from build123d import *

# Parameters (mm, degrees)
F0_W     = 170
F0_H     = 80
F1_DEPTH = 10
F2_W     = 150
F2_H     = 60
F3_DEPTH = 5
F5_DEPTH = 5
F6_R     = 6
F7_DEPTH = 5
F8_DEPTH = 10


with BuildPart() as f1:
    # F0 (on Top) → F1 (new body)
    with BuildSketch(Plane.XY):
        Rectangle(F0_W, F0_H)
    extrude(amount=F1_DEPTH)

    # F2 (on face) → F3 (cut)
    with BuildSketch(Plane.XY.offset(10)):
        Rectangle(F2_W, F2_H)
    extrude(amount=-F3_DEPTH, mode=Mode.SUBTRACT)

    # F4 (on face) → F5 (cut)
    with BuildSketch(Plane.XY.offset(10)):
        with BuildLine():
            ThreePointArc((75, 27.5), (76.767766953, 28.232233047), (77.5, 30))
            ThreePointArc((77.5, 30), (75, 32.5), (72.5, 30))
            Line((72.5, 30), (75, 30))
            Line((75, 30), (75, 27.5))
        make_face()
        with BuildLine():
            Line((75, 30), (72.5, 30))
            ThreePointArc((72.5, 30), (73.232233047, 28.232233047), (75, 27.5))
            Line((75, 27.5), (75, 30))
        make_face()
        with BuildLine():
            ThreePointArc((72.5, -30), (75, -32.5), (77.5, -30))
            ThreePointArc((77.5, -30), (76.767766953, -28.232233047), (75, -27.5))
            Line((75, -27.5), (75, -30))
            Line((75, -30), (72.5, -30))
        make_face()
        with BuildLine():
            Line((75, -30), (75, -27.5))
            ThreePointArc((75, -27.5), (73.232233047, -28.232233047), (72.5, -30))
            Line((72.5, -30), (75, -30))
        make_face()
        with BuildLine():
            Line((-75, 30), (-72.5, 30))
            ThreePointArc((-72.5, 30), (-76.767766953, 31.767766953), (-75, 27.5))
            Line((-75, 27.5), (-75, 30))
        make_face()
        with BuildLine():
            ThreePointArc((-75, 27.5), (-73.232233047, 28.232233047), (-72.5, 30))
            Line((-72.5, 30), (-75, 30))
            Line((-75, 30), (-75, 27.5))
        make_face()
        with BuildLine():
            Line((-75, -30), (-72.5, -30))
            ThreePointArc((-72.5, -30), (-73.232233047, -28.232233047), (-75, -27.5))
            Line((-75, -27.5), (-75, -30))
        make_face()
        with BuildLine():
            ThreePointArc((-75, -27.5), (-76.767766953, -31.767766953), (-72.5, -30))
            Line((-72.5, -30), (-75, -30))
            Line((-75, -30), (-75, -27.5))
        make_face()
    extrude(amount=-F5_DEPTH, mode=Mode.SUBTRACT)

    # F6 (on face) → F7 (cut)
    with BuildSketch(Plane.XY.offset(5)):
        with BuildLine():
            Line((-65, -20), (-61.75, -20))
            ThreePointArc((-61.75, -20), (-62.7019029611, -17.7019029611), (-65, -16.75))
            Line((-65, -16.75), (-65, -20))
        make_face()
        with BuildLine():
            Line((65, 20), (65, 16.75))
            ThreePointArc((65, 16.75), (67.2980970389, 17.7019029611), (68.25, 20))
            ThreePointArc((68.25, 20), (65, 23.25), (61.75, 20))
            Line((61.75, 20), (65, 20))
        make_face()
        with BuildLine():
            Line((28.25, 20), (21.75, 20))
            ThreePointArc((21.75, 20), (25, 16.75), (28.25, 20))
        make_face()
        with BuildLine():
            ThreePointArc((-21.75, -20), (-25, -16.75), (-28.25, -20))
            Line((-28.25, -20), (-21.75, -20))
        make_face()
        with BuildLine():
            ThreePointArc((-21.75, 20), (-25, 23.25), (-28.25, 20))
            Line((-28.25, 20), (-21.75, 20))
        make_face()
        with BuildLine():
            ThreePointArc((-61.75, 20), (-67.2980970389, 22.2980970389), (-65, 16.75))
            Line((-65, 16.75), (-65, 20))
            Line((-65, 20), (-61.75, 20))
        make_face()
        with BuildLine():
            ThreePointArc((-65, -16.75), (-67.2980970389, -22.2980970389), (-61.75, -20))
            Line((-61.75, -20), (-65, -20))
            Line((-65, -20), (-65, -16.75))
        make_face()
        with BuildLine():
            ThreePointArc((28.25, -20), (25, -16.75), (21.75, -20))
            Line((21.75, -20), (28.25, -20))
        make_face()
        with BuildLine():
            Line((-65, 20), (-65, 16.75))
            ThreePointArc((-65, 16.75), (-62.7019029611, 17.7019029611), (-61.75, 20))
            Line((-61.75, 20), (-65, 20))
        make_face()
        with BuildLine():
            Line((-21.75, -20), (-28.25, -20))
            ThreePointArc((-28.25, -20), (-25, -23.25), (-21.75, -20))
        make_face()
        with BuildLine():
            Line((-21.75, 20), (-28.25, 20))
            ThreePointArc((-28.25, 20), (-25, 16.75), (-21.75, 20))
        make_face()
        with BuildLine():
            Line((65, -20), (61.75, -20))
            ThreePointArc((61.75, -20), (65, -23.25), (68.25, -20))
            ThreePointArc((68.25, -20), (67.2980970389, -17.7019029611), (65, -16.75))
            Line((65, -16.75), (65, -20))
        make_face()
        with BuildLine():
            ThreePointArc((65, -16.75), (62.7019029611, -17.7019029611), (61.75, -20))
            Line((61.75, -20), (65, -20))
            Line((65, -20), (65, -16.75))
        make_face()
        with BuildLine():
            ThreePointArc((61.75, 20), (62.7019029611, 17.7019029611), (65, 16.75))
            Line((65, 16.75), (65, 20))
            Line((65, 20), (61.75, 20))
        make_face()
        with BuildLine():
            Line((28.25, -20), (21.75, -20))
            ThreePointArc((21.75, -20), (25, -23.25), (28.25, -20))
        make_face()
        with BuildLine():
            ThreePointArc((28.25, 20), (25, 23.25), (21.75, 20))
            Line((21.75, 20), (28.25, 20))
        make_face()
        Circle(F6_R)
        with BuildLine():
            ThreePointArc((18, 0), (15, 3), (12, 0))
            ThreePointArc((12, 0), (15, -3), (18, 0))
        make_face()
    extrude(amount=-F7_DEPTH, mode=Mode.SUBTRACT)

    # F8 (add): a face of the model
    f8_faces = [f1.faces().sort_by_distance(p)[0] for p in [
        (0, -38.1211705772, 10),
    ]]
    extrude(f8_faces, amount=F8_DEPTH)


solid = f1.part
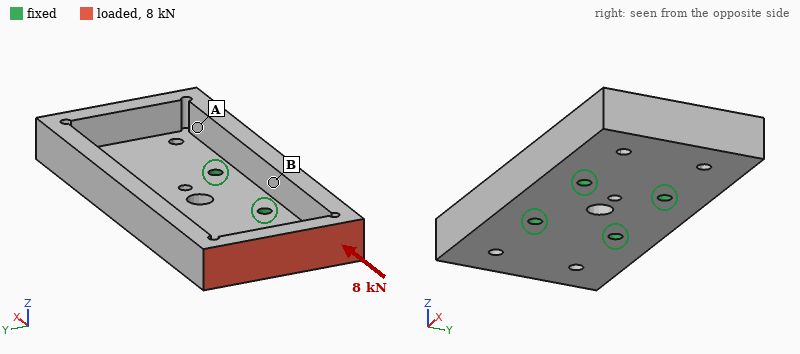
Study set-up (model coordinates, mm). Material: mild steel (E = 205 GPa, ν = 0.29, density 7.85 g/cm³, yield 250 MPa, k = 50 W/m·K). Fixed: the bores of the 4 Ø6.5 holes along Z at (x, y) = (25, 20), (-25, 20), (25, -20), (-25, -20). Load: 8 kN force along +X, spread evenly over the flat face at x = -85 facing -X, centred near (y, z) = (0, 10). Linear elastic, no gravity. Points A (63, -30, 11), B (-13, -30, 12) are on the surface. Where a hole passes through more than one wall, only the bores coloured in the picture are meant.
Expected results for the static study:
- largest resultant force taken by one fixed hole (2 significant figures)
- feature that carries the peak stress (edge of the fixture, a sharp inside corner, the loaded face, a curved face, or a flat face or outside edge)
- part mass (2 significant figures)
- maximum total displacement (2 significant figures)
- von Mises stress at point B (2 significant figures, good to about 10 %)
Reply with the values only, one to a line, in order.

2.7 kN
a curved face
1.1 kg
47 µm
14 MPa
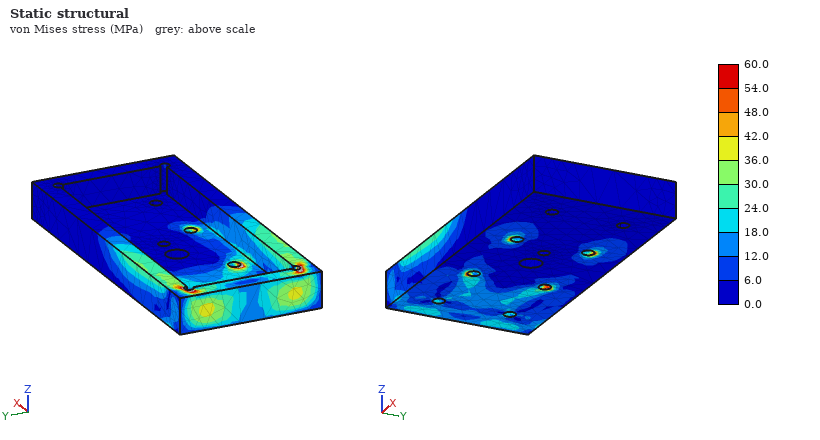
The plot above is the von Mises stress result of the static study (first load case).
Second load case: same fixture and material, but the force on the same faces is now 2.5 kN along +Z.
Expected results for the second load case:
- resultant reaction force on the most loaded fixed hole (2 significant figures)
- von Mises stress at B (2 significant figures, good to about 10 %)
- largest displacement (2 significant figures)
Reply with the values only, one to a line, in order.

3.1 kN
37 MPa
0.11 mm
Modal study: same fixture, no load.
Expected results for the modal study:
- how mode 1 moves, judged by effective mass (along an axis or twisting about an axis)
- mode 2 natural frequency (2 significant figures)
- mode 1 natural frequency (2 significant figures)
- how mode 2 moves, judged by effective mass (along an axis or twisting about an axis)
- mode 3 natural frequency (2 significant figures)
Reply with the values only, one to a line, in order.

twisting about Y
2100 Hz
1700 Hz
along Z
2300 Hz
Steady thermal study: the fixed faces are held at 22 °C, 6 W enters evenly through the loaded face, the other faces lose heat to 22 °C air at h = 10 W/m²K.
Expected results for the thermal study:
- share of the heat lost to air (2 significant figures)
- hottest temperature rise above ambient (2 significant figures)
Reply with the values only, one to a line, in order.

18 %
12 K
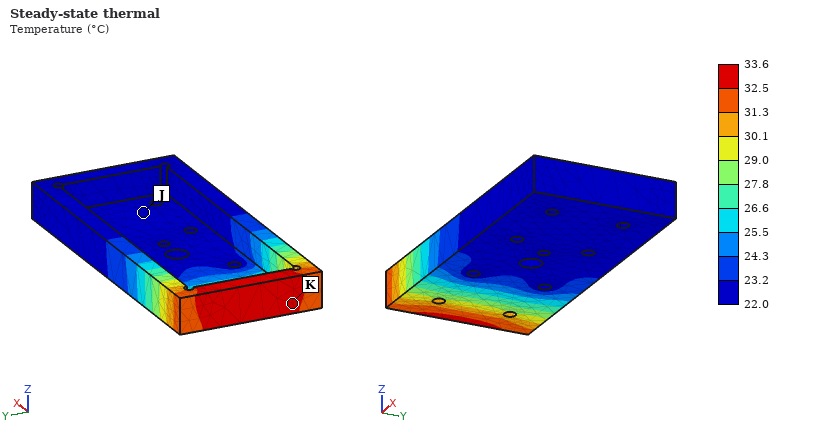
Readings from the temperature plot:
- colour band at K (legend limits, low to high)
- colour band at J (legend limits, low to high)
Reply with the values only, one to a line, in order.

32.5 to 33.6 °C
22.0 to 23.2 °C
